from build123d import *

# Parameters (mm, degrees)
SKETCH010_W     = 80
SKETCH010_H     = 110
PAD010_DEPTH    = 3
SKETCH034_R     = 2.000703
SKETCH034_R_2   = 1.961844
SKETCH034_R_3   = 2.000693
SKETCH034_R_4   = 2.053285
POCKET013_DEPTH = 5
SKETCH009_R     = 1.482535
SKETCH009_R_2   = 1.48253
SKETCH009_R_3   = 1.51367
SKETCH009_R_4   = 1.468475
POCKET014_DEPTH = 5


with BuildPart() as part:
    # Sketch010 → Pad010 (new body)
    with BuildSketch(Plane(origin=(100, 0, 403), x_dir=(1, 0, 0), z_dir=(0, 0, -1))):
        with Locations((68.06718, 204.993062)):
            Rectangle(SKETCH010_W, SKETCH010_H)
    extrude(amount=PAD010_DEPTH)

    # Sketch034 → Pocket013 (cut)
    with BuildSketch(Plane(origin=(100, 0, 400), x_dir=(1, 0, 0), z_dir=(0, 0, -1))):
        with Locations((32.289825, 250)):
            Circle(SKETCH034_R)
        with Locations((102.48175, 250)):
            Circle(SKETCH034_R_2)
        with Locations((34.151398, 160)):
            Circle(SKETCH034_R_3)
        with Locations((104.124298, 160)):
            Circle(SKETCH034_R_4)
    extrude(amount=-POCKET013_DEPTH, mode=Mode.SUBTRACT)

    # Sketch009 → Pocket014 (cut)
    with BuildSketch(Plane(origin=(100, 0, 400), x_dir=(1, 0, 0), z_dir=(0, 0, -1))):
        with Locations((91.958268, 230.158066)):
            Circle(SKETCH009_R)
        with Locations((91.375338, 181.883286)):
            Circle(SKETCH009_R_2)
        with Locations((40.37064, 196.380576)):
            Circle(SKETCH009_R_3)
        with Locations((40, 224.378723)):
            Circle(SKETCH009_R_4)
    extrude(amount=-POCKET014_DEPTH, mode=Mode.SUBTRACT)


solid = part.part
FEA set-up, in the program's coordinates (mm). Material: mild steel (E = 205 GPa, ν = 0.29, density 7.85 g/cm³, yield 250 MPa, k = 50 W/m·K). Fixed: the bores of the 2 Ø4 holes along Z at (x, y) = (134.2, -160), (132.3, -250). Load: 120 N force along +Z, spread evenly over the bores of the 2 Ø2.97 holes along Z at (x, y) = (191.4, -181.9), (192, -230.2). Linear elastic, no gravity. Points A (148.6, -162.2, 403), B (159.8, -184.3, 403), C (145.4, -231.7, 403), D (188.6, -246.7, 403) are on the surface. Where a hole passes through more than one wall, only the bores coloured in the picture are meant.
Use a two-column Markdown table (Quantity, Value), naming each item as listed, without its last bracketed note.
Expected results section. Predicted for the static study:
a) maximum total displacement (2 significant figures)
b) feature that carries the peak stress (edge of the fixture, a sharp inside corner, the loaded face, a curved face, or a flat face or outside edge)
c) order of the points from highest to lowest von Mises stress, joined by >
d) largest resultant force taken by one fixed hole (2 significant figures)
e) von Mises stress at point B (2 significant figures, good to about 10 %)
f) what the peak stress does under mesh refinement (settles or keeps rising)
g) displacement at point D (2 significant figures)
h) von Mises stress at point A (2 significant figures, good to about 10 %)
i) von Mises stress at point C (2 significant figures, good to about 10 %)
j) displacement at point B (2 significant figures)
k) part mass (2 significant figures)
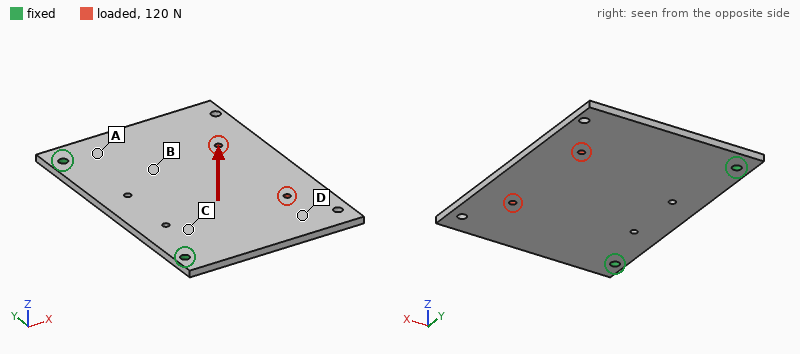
| Quantity | Value |
|---|---|
| maximum total displacement | 0.39 mm |
| feature that carries the peak stress | edge of the fixture |
| order of the points from highest to lowest von Mises stress, joined by > | A > C > B > D |
| largest resultant force taken by one fixed hole | 61 N |
| von Mises stress at point B | 23 MPa |
| what the peak stress does under mesh refinement | keeps rising |
| displacement at point D | 0.25 mm |
| von Mises stress at point A | 43 MPa |
| von Mises stress at point C | 31 MPa |
| displacement at point B | 0.099 mm |
| part mass | 210 g |
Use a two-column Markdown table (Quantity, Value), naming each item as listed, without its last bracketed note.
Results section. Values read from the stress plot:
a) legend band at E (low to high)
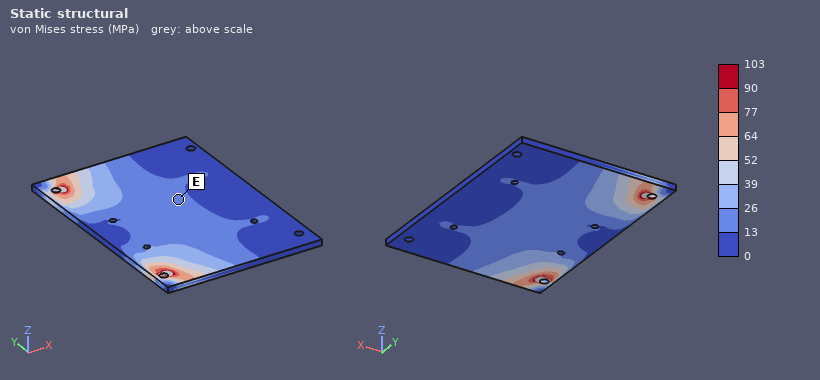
| Quantity | Value |
|---|---|
| legend band at E | 13 to 26 MPa |
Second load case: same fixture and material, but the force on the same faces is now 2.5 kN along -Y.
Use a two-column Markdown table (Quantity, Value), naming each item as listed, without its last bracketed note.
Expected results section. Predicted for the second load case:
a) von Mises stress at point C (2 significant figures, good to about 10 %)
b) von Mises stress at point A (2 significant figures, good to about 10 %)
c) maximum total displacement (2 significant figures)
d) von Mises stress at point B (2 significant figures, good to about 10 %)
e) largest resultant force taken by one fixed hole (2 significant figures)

| Quantity | Value |
|---|---|
| von Mises stress at point C | 19 MPa |
| von Mises stress at point A | 23 MPa |
| maximum total displacement | 15 µm |
| von Mises stress at point B | 17 MPa |
| largest resultant force taken by one fixed hole | 2.1 kN |
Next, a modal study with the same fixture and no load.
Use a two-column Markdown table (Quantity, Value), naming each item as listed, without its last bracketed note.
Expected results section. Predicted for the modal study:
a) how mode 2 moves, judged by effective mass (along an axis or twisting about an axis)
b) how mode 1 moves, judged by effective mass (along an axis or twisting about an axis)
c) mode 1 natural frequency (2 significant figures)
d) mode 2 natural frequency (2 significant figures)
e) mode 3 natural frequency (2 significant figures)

| Quantity | Value |
|---|---|
| how mode 2 moves, judged by effective mass | twisting about X |
| how mode 1 moves, judged by effective mass | along Z |
| mode 1 natural frequency | 340 Hz |
| mode 2 natural frequency | 830 Hz |
| mode 3 natural frequency | 1600 Hz |
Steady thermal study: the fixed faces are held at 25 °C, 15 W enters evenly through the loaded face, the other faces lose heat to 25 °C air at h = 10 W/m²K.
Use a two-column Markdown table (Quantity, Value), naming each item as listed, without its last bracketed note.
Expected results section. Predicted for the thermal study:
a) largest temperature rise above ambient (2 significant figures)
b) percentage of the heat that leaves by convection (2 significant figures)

| Quantity | Value |
|---|---|
| largest temperature rise above ambient | 67 K |
| percentage of the heat that leaves by convection | 42 % |
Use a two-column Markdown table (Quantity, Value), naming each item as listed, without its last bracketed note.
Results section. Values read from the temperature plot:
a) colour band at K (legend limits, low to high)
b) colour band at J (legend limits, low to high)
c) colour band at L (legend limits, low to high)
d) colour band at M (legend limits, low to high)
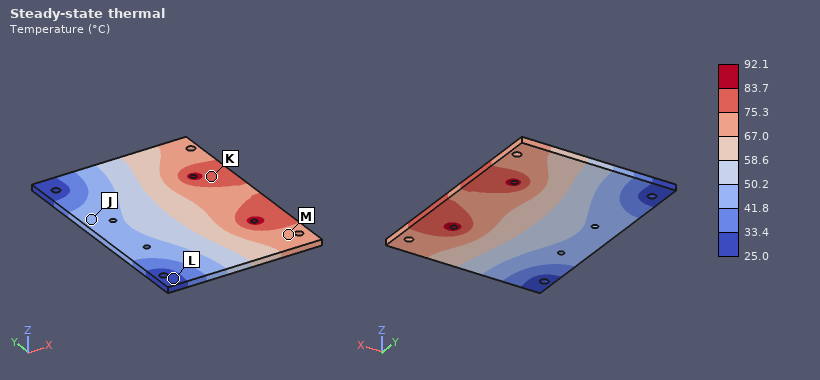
| Quantity | Value |
|---|---|
| colour band at K | 75.3 to 83.7 °C |
| colour band at J | 41.8 to 50.2 °C |
| colour band at L | 25.0 to 33.4 °C |
| colour band at M | 67.0 to 75.3 °C |
